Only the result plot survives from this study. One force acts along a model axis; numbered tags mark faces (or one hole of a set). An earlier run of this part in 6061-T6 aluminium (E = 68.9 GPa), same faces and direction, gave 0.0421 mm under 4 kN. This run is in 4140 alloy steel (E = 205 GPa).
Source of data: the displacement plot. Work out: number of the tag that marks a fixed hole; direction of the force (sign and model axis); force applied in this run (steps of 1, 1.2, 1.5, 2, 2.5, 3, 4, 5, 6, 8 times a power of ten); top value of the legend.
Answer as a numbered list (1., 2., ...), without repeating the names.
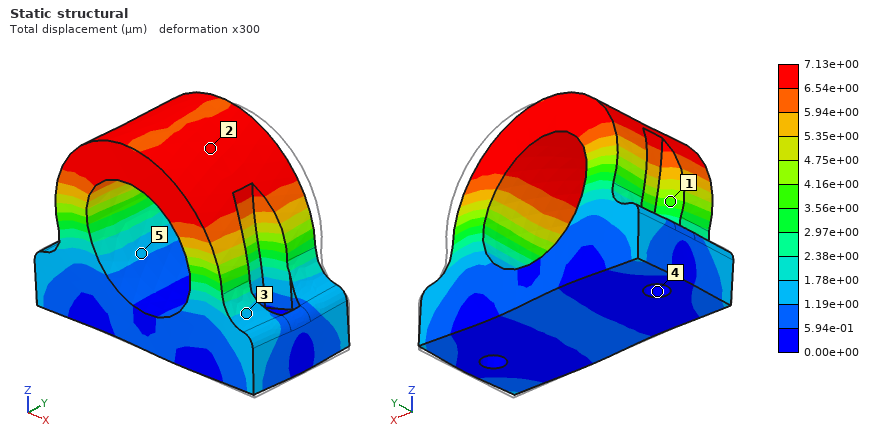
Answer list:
1. 4
2. -X
3. 2 kN
4. 7.13e+00 µm
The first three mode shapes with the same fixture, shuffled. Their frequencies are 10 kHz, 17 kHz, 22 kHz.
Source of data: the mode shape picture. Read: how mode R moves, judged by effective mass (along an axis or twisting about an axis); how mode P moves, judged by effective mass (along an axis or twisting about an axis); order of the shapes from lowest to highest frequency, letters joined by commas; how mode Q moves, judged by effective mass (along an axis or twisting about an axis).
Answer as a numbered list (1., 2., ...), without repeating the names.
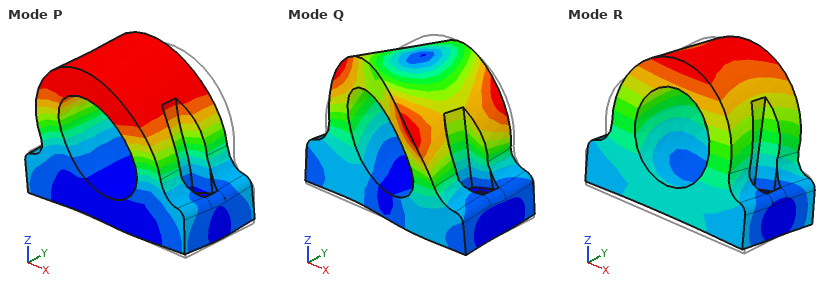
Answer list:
1. along Y
2. along X
3. R, P, Q
4. twisting about Z
